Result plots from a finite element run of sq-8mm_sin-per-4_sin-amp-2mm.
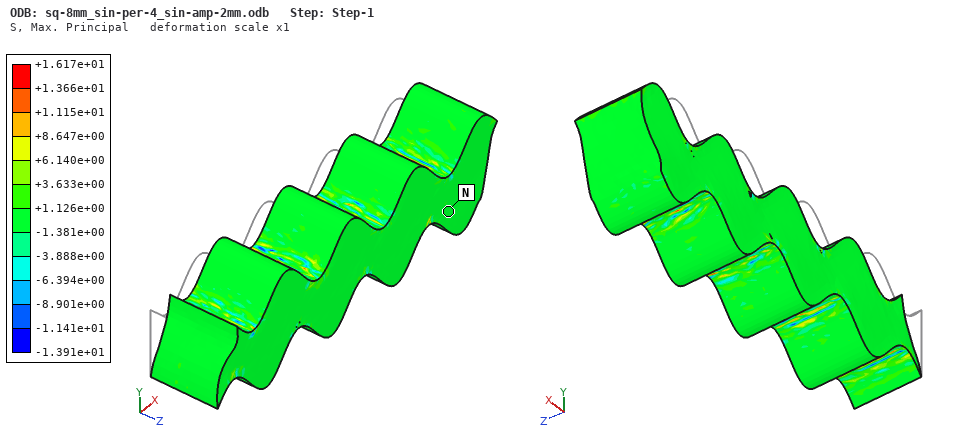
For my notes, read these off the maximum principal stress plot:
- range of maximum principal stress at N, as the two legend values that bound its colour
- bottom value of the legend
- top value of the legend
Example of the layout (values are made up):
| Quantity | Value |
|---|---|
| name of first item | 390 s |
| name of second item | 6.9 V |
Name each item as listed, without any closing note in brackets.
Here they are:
| Quantity | Value |
|---|---|
| range of maximum principal stress at N, as the two legend values that bound its colour | -1.381e+00 to +1.126e+00 |
| bottom value of the legend | -1.391e+01 |
| top value of the legend | +1.617e+01 |
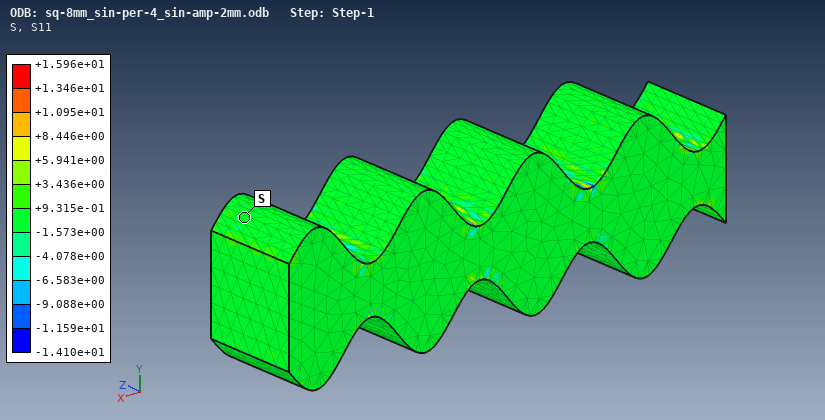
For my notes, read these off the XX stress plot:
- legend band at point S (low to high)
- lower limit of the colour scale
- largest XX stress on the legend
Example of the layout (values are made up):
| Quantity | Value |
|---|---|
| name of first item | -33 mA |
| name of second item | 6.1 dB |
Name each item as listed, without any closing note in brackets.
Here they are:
| Quantity | Value |
|---|---|
| legend band at point S | -1.573e+00 to +9.315e-01 |
| lower limit of the colour scale | -1.410e+01 |
| largest XX stress on the legend | +1.596e+01 |
